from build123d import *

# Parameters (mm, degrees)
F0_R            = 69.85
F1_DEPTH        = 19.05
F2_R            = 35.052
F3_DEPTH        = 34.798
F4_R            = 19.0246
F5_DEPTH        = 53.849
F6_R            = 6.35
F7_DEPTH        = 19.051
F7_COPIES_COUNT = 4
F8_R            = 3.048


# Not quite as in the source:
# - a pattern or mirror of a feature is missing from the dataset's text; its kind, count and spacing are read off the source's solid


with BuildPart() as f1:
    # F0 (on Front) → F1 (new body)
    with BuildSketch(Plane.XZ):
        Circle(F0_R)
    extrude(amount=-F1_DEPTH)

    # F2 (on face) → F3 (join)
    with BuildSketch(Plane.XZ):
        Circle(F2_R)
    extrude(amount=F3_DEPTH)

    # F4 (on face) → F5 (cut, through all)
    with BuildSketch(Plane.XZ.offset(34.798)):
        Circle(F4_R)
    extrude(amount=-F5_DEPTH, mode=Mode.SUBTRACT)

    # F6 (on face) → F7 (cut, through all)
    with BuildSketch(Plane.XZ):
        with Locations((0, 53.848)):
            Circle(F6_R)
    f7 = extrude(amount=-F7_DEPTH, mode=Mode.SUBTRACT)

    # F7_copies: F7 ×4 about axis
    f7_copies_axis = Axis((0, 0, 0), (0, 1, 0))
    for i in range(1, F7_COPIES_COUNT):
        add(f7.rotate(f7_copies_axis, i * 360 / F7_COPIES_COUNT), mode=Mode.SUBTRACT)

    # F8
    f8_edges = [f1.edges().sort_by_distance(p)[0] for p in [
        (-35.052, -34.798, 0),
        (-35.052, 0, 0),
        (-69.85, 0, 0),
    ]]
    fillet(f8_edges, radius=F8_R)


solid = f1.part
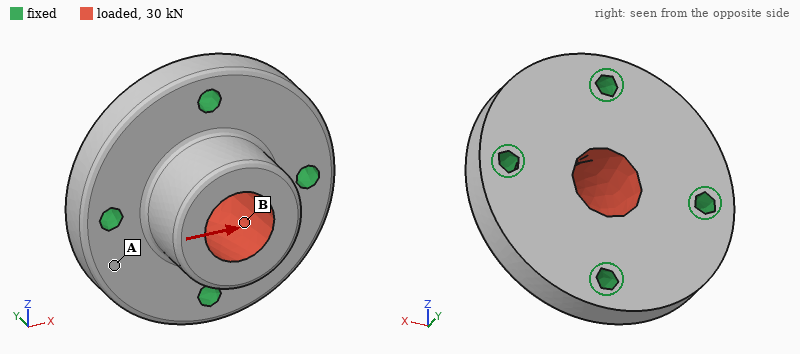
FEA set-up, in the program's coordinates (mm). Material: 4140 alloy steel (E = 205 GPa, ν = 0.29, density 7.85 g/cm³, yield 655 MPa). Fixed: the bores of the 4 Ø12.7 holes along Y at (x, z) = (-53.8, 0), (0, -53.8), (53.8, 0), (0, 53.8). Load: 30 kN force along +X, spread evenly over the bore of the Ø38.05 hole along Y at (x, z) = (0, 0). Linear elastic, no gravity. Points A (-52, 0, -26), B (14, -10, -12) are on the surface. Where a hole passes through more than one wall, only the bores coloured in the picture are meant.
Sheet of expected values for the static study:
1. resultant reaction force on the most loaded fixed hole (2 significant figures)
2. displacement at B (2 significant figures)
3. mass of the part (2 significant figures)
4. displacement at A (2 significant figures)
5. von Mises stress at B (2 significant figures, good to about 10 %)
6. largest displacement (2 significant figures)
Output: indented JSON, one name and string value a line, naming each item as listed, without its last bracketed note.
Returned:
{
  "resultant reaction force on the most loaded fixed hole": "11 kN",
  "displacement at B": "4.2 µm",
  "mass of the part": "2.8 kg",
  "displacement at A": "1.5 µm",
  "von Mises stress at B": "14 MPa",
  "largest displacement": "8.4 µm"
}
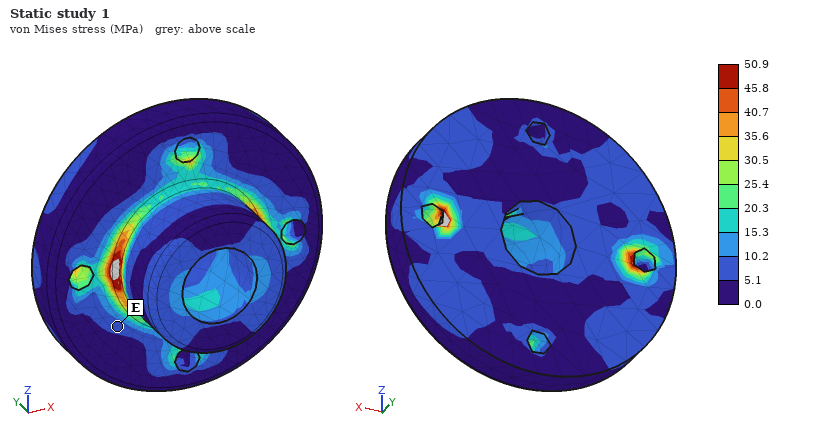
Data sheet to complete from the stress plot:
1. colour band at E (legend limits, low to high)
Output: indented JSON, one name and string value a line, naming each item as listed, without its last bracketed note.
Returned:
{
  "colour band at E": "5.1 to 10.2 MPa"
}
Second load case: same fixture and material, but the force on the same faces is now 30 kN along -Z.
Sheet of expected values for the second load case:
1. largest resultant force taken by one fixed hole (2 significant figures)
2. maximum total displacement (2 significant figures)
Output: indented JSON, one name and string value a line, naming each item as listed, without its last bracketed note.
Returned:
{
  "largest resultant force taken by one fixed hole": "11 kN",
  "maximum total displacement": "8.4 µm"
}
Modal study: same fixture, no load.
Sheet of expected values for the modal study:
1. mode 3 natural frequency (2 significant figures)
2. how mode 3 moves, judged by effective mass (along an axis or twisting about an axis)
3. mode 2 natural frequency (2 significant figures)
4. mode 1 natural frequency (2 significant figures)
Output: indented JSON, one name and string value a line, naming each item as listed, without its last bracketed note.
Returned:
{
  "mode 3 natural frequency": "9800 Hz",
  "how mode 3 moves, judged by effective mass": "along Y",
  "mode 2 natural frequency": "9300 Hz",
  "mode 1 natural frequency": "9300 Hz"
}
